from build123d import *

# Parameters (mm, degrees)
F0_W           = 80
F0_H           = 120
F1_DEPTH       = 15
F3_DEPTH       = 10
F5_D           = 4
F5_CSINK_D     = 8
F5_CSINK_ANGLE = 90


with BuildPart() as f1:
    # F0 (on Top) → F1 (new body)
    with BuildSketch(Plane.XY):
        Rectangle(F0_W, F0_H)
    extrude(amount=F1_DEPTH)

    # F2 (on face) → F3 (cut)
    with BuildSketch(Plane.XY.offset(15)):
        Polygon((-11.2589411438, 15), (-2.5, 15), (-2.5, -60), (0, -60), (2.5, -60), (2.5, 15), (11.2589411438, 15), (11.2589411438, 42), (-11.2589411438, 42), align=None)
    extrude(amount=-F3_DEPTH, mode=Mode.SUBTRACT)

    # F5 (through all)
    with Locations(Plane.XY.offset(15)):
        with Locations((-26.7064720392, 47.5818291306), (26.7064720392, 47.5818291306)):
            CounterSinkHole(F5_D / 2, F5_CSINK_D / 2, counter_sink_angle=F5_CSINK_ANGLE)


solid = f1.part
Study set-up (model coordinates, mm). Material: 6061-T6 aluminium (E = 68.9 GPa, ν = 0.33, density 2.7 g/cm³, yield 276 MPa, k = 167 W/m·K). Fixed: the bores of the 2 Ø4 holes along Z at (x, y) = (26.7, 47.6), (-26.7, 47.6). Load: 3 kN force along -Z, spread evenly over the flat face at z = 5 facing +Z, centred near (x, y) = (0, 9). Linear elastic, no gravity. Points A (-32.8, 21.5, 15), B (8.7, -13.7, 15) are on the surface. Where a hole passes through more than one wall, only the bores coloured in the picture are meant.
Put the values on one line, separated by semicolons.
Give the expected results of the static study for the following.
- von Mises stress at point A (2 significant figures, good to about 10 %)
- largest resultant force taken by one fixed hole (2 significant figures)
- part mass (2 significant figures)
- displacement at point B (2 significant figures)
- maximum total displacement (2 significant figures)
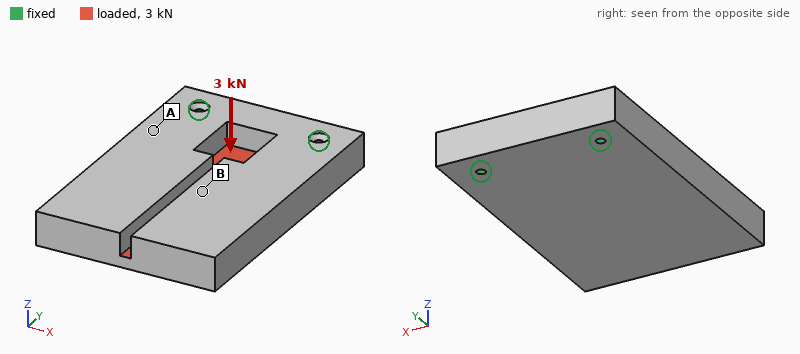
23 MPa; 1.5 kN; 360 g; 0.18 mm; 0.34 mm
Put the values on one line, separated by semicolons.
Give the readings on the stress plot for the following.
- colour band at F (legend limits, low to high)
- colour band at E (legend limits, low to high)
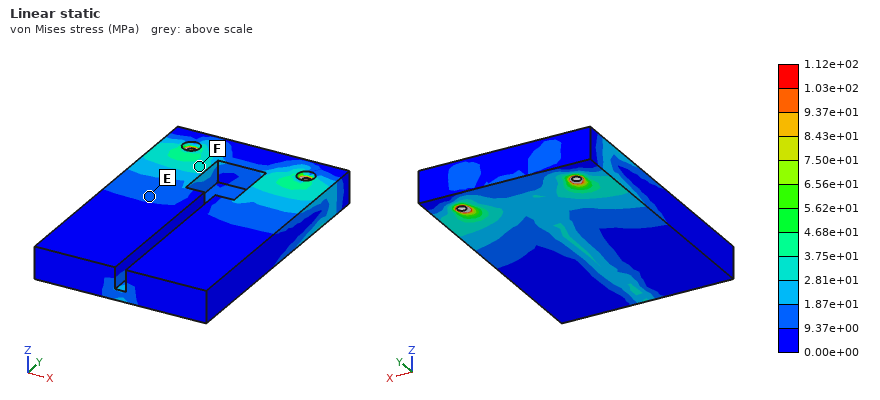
2.81e+01 to 3.75e+01 MPa; 9.37e+00 to 1.87e+01 MPa
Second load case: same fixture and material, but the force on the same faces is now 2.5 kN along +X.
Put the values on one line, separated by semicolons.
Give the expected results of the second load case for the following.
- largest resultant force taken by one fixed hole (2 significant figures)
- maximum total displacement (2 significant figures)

2.1 kN; 16 µm
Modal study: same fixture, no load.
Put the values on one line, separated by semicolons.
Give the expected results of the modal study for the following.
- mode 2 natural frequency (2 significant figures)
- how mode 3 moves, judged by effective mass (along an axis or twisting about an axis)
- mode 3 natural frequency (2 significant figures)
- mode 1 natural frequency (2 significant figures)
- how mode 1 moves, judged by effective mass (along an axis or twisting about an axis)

2500 Hz; along X; 3400 Hz; 840 Hz; along Z
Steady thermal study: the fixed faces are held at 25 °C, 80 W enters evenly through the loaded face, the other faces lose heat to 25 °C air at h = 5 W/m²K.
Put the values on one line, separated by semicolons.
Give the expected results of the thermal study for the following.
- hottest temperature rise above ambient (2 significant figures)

23 K
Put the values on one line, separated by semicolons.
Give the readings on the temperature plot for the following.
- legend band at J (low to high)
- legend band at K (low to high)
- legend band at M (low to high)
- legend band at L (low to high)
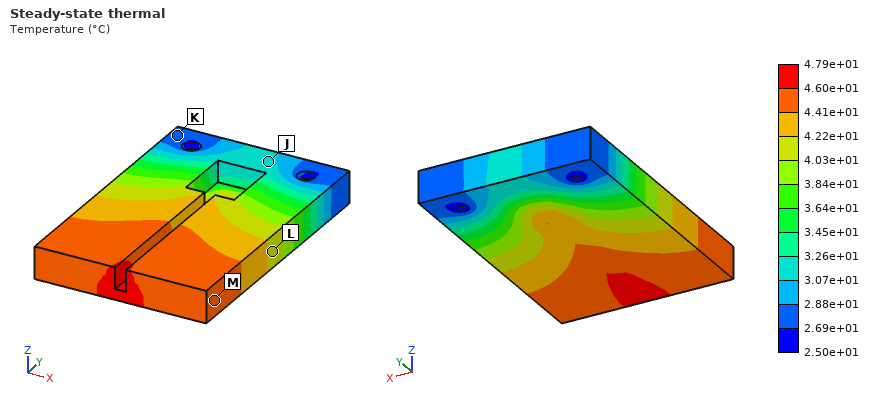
3.07e+01 to 3.26e+01 °C; 2.69e+01 to 2.88e+01 °C; 4.41e+01 to 4.60e+01 °C; 4.03e+01 to 4.22e+01 °C
